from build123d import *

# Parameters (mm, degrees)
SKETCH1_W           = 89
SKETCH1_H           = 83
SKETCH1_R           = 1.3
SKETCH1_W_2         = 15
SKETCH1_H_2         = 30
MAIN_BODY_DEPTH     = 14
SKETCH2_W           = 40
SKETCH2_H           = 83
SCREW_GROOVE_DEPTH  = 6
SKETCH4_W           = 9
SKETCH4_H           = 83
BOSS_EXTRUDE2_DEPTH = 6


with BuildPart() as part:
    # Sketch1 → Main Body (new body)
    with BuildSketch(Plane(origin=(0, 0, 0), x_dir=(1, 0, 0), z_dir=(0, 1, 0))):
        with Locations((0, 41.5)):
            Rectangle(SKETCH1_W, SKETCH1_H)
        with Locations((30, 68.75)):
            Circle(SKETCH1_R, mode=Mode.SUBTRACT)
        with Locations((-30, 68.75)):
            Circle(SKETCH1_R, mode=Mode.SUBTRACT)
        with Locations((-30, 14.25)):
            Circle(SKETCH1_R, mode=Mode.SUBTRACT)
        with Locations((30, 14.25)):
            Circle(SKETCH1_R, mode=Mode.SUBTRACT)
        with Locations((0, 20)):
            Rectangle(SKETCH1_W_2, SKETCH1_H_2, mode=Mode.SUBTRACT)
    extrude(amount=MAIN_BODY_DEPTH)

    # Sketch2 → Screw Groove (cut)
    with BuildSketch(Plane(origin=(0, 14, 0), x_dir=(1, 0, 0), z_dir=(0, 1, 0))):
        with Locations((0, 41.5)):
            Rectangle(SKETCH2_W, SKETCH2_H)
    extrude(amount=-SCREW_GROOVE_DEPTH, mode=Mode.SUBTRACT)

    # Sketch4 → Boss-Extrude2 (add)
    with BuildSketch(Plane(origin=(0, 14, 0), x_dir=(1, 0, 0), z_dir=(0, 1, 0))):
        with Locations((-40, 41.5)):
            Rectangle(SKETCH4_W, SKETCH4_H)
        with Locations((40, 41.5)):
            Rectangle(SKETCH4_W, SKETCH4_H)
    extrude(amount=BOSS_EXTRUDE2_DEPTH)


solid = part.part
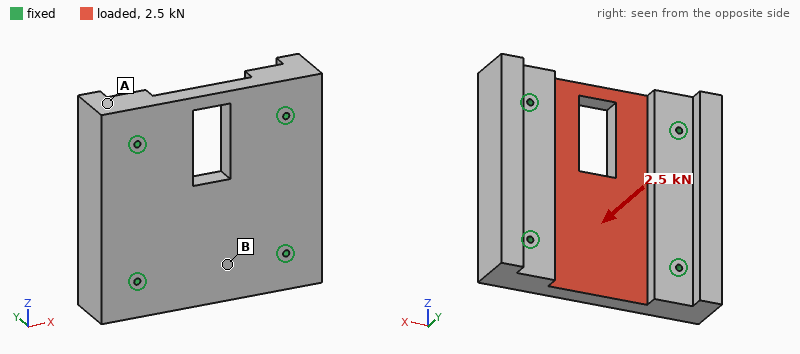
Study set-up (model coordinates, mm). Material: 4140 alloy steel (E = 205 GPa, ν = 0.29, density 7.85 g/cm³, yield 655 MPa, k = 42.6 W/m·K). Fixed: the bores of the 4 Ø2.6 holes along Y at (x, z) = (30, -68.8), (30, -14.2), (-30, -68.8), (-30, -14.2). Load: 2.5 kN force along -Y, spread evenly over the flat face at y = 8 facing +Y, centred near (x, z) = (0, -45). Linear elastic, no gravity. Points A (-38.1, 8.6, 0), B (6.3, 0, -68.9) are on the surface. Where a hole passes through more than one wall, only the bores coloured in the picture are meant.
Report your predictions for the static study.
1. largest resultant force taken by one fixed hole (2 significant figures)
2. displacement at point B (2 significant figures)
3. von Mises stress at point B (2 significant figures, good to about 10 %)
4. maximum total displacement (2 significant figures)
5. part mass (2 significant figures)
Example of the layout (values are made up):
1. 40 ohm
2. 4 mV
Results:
1. 810 N
2. 2.8 µm
3. 9.1 MPa
4. 3.8 µm
5. 700 g
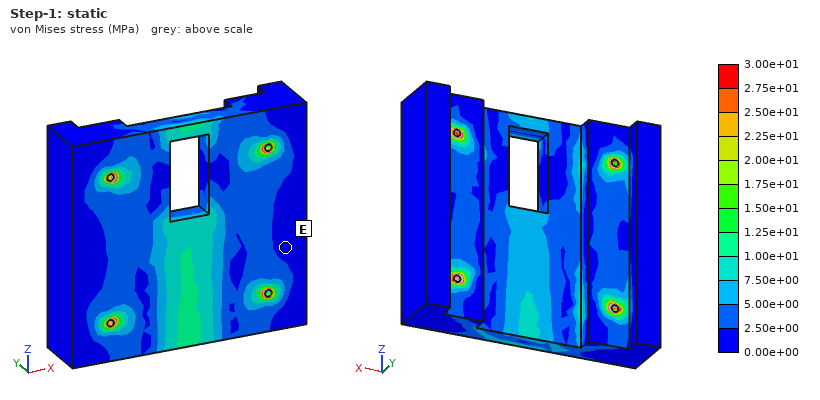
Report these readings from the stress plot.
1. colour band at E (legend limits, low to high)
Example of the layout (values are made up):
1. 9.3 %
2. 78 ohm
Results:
1. 0.00e+00 to 2.50e+00 MPa
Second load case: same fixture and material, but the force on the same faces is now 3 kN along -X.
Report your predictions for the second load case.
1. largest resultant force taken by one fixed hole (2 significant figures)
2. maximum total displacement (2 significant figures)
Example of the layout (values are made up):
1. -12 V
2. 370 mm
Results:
1. 870 N
2. 0.65 µm
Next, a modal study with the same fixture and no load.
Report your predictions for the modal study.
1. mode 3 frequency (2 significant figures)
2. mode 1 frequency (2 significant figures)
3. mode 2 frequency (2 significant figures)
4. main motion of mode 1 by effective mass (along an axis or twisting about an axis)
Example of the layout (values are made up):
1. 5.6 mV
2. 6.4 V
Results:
1. 13 kHz
2. 10 kHz
3. 13 kHz
4. along Y
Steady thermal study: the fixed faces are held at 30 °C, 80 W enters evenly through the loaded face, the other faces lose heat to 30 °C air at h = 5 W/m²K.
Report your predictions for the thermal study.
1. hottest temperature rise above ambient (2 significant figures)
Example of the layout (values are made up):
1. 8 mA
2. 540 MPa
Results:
1. 38 K
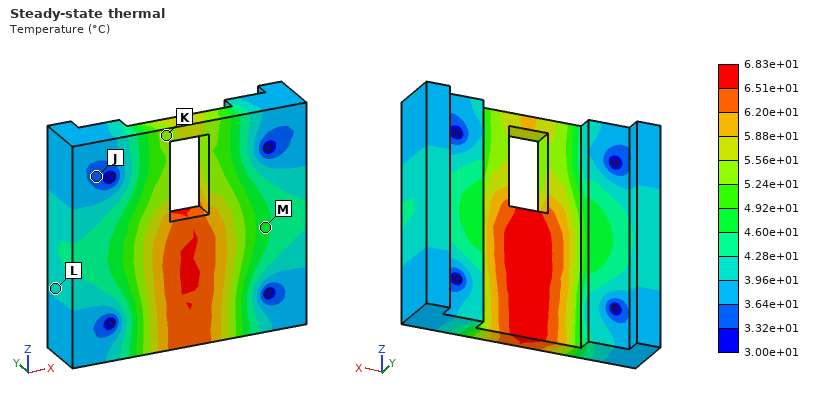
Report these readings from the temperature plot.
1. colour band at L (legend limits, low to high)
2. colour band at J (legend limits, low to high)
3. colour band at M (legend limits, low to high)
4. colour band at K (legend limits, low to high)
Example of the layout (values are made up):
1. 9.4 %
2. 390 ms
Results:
1. 3.96e+01 to 4.28e+01 °C
2. 3.32e+01 to 3.64e+01 °C
3. 4.60e+01 to 4.92e+01 °C
4. 5.24e+01 to 5.56e+01 °C
